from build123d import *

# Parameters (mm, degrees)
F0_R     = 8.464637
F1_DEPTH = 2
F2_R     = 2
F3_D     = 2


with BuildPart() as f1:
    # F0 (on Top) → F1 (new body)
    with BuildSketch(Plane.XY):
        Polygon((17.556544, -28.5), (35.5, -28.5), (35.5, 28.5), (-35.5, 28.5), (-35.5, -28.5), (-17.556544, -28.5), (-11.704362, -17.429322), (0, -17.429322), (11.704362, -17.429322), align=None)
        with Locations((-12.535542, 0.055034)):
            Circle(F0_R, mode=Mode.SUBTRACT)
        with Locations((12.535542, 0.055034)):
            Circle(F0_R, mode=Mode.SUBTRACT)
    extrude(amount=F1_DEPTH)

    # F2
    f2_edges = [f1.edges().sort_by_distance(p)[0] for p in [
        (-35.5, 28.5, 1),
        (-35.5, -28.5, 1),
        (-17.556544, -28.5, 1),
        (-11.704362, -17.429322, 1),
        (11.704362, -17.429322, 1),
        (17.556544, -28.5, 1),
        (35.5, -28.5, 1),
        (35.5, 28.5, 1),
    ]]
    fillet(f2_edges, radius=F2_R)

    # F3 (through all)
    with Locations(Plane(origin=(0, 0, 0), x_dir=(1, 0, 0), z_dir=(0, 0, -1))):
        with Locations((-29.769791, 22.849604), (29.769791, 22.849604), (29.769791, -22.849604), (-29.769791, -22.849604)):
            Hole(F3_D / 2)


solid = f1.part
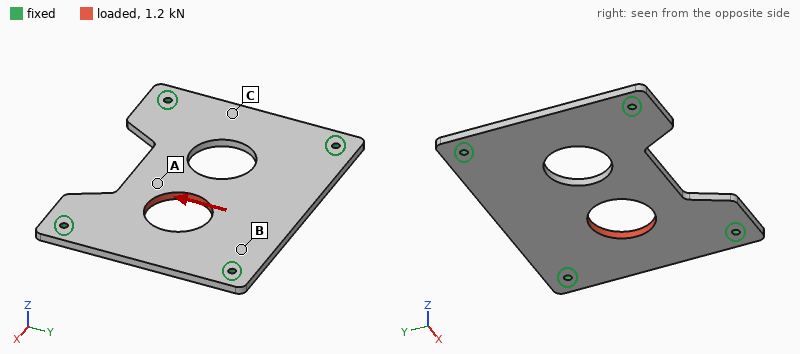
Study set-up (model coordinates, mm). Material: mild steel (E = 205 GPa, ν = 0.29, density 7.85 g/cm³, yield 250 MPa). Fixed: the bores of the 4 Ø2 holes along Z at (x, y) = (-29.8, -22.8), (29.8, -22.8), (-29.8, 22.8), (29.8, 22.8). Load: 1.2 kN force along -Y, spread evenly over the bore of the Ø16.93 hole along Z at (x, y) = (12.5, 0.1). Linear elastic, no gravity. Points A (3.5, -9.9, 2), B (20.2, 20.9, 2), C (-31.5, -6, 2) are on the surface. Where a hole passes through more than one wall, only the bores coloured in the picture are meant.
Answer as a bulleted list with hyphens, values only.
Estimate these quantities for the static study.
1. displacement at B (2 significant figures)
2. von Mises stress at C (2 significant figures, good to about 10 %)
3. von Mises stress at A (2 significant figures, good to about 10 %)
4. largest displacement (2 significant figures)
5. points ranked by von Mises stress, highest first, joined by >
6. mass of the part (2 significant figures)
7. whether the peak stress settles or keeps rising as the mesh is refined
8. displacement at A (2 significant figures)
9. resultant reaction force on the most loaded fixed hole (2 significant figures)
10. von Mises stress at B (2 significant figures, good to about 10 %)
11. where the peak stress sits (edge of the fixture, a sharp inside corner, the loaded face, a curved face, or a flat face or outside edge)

- 1.8 µm
- 3.4 MPa
- 8.3 MPa
- 4.0 µm
- B > A > C
- 51 g
- keeps rising
- 3.7 µm
- 490 N
- 12 MPa
- edge of the fixture
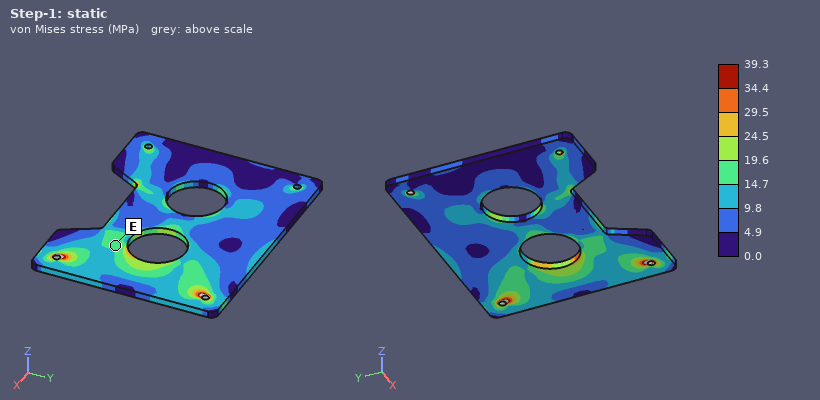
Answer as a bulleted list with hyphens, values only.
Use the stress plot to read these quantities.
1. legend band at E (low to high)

- 14.7 to 19.6 MPa
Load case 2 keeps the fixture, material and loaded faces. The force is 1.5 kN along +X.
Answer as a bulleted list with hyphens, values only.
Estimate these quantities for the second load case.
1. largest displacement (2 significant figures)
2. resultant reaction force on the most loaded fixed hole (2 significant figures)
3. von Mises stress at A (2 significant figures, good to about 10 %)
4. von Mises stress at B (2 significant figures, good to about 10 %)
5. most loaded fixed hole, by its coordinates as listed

- 4.5 µm
- 510 N
- 20 MPa
- 14 MPa
- (29.8, 22.8)
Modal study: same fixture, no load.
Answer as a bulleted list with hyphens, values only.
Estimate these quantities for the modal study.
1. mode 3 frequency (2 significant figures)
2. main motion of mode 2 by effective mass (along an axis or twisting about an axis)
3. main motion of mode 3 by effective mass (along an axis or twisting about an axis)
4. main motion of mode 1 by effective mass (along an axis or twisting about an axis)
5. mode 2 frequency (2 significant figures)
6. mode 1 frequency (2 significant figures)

- 4800 Hz
- twisting about X
- twisting about Y
- along Z
- 3600 Hz
- 2400 Hz
